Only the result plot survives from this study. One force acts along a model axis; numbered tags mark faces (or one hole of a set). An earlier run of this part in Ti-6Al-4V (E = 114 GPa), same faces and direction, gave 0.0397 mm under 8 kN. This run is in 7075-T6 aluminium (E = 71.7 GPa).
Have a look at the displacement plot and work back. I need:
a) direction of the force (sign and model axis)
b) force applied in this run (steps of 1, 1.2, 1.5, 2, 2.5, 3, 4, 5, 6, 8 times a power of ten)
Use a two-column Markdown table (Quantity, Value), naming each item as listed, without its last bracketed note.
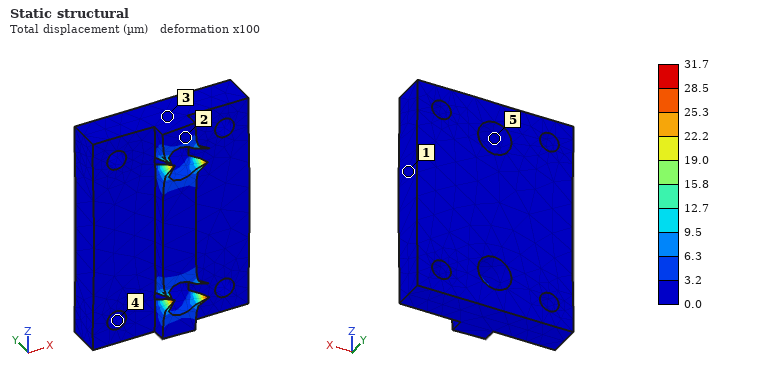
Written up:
| Quantity | Value |
|---|---|
| direction of the force | +X |
| force applied in this run | 4 kN |
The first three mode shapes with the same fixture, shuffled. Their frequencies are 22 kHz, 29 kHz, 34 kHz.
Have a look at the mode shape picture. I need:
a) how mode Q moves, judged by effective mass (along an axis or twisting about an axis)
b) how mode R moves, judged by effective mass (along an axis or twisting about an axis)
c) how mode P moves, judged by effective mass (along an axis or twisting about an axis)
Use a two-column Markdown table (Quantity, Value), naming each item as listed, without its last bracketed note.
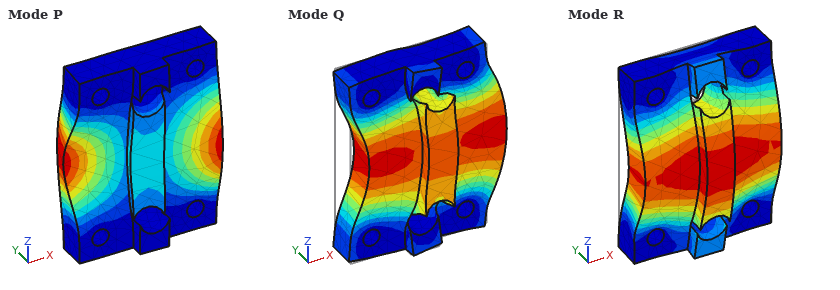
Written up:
| Quantity | Value |
|---|---|
| how mode Q moves, judged by effective mass | along X |
| how mode R moves, judged by effective mass | along Y |
| how mode P moves, judged by effective mass | twisting about Z |
